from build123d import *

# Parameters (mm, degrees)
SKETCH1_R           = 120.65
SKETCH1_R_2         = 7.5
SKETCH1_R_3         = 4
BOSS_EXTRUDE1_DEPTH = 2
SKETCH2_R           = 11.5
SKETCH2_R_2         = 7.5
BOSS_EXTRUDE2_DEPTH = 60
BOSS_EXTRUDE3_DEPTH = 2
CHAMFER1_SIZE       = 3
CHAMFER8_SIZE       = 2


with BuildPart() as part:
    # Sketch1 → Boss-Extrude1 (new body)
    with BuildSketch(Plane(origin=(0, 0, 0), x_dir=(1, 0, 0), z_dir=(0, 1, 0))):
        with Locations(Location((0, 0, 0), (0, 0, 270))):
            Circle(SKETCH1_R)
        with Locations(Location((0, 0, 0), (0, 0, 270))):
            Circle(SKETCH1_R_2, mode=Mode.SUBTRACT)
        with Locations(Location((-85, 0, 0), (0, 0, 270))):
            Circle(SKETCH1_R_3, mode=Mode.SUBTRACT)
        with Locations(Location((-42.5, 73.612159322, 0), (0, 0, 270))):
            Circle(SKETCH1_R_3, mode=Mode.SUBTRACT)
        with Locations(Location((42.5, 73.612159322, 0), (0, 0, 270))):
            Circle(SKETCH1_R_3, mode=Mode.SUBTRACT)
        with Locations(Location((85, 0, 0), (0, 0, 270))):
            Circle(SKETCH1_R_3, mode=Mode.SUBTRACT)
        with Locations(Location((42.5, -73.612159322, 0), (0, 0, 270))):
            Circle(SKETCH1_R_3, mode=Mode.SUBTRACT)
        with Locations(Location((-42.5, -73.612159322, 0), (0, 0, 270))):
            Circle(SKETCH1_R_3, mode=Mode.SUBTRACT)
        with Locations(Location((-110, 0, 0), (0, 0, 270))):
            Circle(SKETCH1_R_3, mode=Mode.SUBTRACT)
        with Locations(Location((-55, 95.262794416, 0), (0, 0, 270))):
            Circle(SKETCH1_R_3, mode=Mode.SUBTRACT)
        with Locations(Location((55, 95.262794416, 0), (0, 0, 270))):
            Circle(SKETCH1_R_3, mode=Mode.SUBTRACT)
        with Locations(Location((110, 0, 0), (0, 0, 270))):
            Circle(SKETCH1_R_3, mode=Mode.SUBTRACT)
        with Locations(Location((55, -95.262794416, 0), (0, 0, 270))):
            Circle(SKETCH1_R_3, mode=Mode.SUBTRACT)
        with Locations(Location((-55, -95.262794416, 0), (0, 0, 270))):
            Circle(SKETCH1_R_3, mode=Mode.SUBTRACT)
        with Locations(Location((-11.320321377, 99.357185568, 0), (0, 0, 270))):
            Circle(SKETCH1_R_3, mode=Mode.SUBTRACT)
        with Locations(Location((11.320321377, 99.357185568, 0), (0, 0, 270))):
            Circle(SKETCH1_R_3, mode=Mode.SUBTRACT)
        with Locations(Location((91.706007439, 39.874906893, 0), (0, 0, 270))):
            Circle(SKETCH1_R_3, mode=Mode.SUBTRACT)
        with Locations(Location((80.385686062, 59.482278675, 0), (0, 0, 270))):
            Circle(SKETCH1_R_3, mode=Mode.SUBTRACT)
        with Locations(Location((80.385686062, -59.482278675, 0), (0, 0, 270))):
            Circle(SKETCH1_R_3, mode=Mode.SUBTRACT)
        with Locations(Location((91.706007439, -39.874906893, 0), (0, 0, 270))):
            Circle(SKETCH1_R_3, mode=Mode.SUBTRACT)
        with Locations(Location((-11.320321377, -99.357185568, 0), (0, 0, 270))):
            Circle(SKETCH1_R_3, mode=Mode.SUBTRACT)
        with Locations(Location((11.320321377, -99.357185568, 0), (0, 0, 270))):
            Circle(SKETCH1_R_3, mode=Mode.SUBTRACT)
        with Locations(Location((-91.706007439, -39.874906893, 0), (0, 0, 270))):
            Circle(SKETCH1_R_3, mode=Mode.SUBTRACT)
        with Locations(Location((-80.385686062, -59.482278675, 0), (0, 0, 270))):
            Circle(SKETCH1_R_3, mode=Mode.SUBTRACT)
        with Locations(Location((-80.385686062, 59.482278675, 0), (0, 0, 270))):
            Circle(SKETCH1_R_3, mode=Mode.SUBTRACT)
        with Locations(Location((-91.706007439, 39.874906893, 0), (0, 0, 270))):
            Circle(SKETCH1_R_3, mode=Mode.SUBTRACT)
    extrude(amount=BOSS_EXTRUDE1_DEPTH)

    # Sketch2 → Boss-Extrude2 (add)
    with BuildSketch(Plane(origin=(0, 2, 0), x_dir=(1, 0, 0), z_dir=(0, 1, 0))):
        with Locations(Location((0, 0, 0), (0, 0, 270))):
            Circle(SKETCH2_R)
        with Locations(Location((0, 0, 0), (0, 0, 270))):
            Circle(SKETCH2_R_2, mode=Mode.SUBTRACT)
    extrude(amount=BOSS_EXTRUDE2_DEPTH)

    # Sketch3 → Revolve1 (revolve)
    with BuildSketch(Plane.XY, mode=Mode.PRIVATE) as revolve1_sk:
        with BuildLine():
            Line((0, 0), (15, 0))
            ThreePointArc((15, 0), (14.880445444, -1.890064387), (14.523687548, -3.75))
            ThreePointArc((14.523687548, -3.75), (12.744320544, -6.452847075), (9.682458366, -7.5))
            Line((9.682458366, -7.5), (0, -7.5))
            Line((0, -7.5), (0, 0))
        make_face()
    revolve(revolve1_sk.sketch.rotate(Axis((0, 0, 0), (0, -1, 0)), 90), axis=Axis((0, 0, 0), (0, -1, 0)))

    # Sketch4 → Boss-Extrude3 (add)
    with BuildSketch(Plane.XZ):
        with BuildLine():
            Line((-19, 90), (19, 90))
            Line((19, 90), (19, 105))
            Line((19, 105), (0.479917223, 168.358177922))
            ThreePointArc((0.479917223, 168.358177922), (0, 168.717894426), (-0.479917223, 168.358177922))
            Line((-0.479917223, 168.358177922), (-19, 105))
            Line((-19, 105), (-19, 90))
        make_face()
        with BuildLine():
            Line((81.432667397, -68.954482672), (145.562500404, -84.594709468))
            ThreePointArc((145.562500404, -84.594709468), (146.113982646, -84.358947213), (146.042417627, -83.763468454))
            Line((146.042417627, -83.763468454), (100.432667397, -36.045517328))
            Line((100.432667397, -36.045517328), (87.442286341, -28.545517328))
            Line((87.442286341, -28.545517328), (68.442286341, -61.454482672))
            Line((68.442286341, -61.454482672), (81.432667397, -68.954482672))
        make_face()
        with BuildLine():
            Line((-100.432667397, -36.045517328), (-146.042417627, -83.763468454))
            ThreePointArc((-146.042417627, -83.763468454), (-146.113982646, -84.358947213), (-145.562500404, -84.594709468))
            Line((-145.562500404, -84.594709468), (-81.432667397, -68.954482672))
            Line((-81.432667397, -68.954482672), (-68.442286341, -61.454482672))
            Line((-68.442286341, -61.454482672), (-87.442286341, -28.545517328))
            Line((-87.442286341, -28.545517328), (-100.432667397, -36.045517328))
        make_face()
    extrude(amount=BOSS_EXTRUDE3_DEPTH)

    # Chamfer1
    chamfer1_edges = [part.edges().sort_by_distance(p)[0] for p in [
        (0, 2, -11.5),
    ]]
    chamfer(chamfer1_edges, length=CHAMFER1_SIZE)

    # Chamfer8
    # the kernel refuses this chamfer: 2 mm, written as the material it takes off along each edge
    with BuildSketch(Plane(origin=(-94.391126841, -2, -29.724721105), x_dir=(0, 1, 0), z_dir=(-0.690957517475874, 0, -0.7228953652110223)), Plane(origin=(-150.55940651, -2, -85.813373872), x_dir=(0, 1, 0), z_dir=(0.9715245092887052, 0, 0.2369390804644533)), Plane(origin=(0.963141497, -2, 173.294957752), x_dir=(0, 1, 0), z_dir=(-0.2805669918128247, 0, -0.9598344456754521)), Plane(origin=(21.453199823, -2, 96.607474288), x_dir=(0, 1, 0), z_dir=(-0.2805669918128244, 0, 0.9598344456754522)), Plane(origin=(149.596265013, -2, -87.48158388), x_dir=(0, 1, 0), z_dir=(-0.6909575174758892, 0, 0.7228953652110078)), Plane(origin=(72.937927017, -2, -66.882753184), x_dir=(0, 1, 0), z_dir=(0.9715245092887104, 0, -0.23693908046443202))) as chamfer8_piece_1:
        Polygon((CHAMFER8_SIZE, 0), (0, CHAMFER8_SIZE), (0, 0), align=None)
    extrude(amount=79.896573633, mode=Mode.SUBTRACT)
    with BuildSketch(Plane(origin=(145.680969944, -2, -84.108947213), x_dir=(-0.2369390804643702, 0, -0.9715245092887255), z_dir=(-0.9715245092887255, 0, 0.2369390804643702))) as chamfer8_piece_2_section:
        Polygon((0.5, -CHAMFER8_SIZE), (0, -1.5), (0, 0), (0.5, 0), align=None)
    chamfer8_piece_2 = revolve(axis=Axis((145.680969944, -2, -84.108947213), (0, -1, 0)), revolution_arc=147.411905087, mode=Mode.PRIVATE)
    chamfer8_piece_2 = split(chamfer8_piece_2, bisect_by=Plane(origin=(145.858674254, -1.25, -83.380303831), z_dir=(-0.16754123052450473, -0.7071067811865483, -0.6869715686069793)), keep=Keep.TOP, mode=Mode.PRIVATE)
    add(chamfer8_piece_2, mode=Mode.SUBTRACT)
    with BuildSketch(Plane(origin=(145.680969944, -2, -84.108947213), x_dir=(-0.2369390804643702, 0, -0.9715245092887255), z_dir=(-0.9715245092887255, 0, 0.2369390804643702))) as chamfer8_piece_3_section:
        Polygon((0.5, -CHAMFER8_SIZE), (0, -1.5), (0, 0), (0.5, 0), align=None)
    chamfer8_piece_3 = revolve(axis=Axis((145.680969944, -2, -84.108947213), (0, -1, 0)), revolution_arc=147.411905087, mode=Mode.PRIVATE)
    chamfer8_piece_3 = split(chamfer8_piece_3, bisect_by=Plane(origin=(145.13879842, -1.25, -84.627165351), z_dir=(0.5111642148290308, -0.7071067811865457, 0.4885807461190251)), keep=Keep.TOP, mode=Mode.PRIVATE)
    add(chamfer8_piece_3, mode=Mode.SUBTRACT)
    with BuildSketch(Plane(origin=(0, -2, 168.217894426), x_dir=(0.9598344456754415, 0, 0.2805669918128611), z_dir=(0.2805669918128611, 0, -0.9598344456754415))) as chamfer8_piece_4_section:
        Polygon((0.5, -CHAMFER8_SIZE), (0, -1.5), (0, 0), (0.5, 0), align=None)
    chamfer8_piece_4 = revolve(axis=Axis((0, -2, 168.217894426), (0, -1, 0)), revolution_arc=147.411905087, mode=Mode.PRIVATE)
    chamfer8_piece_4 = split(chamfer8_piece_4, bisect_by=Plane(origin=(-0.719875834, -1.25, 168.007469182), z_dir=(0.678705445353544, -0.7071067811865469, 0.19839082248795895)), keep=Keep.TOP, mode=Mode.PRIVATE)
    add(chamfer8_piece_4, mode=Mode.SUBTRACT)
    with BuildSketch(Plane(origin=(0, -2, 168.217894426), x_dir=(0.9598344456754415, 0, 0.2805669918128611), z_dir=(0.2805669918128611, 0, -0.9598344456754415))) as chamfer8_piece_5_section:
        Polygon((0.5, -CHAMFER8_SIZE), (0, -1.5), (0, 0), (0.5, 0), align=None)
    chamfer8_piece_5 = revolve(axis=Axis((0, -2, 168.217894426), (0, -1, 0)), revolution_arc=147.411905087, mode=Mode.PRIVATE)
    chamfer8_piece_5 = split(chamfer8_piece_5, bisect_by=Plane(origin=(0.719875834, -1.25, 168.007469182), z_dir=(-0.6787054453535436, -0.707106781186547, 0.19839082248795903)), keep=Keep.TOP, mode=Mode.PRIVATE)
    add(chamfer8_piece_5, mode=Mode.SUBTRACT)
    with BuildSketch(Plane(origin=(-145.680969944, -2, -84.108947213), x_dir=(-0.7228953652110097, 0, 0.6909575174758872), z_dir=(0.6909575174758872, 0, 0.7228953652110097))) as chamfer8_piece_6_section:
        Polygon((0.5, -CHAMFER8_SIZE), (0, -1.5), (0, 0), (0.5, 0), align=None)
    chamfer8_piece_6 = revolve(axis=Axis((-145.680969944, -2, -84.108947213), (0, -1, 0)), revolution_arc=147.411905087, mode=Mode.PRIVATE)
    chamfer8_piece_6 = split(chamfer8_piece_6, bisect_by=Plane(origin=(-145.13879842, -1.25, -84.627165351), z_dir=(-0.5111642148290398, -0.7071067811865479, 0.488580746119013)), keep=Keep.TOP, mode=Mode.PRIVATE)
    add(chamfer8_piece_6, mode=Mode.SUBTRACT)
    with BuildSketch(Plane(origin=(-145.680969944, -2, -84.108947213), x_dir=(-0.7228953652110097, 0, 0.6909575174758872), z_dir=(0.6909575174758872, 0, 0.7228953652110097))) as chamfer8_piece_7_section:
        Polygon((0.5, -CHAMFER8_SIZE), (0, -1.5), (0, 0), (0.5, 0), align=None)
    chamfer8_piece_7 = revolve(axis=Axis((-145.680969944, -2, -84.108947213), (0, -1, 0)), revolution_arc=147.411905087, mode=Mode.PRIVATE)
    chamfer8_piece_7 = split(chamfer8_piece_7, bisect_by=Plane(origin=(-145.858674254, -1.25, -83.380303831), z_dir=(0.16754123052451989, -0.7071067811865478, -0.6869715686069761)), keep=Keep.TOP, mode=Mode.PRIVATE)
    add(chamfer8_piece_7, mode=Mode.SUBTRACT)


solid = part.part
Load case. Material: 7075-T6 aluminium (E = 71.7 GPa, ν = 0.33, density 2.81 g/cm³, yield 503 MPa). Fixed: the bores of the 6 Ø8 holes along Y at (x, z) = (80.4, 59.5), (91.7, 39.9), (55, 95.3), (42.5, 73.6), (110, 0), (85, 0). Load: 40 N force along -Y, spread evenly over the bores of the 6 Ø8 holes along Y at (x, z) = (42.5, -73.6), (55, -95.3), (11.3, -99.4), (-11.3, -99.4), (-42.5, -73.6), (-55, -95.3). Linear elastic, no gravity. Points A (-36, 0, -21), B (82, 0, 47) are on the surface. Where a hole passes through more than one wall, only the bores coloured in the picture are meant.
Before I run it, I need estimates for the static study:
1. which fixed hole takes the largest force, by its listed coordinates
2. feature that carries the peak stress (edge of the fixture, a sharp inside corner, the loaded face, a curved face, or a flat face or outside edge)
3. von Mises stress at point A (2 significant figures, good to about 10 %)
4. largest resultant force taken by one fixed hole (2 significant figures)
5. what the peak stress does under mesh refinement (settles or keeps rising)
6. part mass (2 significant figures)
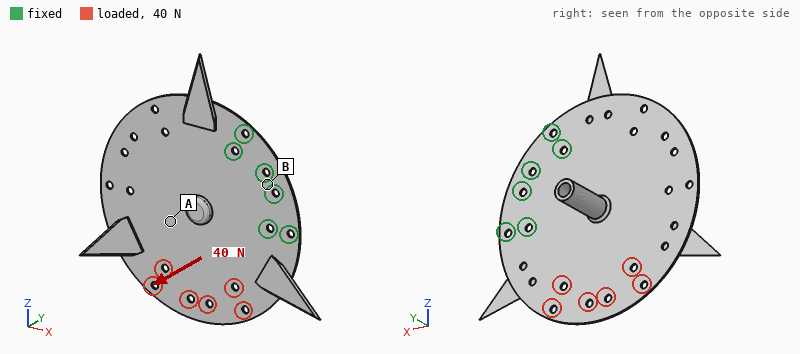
(85, 0)
edge of the fixture
12 MPa
110 N
keeps rising
330 g
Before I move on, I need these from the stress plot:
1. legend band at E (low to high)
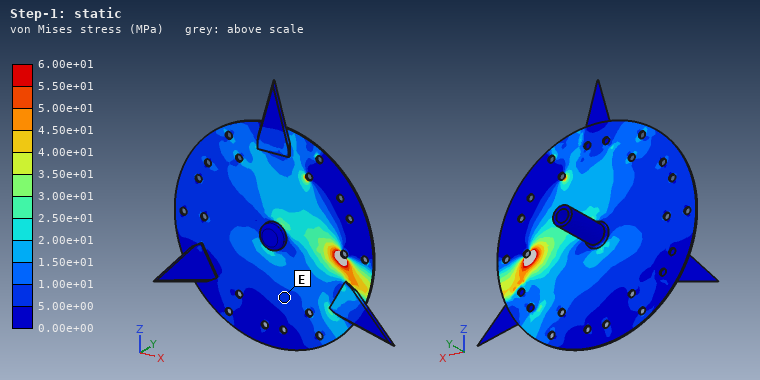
5.00e+00 to 1.00e+01 MPa
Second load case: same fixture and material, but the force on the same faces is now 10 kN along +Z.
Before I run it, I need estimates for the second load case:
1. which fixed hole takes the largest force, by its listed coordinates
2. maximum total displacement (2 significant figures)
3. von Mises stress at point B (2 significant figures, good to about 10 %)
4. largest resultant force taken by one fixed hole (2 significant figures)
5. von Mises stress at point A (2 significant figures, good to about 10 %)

(42.5, 73.6)
0.34 mm
14 MPa
6.5 kN
31 MPa
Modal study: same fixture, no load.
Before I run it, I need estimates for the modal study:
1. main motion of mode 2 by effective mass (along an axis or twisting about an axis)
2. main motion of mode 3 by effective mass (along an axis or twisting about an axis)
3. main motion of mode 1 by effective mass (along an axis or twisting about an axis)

twisting about X
along Y
along Y
